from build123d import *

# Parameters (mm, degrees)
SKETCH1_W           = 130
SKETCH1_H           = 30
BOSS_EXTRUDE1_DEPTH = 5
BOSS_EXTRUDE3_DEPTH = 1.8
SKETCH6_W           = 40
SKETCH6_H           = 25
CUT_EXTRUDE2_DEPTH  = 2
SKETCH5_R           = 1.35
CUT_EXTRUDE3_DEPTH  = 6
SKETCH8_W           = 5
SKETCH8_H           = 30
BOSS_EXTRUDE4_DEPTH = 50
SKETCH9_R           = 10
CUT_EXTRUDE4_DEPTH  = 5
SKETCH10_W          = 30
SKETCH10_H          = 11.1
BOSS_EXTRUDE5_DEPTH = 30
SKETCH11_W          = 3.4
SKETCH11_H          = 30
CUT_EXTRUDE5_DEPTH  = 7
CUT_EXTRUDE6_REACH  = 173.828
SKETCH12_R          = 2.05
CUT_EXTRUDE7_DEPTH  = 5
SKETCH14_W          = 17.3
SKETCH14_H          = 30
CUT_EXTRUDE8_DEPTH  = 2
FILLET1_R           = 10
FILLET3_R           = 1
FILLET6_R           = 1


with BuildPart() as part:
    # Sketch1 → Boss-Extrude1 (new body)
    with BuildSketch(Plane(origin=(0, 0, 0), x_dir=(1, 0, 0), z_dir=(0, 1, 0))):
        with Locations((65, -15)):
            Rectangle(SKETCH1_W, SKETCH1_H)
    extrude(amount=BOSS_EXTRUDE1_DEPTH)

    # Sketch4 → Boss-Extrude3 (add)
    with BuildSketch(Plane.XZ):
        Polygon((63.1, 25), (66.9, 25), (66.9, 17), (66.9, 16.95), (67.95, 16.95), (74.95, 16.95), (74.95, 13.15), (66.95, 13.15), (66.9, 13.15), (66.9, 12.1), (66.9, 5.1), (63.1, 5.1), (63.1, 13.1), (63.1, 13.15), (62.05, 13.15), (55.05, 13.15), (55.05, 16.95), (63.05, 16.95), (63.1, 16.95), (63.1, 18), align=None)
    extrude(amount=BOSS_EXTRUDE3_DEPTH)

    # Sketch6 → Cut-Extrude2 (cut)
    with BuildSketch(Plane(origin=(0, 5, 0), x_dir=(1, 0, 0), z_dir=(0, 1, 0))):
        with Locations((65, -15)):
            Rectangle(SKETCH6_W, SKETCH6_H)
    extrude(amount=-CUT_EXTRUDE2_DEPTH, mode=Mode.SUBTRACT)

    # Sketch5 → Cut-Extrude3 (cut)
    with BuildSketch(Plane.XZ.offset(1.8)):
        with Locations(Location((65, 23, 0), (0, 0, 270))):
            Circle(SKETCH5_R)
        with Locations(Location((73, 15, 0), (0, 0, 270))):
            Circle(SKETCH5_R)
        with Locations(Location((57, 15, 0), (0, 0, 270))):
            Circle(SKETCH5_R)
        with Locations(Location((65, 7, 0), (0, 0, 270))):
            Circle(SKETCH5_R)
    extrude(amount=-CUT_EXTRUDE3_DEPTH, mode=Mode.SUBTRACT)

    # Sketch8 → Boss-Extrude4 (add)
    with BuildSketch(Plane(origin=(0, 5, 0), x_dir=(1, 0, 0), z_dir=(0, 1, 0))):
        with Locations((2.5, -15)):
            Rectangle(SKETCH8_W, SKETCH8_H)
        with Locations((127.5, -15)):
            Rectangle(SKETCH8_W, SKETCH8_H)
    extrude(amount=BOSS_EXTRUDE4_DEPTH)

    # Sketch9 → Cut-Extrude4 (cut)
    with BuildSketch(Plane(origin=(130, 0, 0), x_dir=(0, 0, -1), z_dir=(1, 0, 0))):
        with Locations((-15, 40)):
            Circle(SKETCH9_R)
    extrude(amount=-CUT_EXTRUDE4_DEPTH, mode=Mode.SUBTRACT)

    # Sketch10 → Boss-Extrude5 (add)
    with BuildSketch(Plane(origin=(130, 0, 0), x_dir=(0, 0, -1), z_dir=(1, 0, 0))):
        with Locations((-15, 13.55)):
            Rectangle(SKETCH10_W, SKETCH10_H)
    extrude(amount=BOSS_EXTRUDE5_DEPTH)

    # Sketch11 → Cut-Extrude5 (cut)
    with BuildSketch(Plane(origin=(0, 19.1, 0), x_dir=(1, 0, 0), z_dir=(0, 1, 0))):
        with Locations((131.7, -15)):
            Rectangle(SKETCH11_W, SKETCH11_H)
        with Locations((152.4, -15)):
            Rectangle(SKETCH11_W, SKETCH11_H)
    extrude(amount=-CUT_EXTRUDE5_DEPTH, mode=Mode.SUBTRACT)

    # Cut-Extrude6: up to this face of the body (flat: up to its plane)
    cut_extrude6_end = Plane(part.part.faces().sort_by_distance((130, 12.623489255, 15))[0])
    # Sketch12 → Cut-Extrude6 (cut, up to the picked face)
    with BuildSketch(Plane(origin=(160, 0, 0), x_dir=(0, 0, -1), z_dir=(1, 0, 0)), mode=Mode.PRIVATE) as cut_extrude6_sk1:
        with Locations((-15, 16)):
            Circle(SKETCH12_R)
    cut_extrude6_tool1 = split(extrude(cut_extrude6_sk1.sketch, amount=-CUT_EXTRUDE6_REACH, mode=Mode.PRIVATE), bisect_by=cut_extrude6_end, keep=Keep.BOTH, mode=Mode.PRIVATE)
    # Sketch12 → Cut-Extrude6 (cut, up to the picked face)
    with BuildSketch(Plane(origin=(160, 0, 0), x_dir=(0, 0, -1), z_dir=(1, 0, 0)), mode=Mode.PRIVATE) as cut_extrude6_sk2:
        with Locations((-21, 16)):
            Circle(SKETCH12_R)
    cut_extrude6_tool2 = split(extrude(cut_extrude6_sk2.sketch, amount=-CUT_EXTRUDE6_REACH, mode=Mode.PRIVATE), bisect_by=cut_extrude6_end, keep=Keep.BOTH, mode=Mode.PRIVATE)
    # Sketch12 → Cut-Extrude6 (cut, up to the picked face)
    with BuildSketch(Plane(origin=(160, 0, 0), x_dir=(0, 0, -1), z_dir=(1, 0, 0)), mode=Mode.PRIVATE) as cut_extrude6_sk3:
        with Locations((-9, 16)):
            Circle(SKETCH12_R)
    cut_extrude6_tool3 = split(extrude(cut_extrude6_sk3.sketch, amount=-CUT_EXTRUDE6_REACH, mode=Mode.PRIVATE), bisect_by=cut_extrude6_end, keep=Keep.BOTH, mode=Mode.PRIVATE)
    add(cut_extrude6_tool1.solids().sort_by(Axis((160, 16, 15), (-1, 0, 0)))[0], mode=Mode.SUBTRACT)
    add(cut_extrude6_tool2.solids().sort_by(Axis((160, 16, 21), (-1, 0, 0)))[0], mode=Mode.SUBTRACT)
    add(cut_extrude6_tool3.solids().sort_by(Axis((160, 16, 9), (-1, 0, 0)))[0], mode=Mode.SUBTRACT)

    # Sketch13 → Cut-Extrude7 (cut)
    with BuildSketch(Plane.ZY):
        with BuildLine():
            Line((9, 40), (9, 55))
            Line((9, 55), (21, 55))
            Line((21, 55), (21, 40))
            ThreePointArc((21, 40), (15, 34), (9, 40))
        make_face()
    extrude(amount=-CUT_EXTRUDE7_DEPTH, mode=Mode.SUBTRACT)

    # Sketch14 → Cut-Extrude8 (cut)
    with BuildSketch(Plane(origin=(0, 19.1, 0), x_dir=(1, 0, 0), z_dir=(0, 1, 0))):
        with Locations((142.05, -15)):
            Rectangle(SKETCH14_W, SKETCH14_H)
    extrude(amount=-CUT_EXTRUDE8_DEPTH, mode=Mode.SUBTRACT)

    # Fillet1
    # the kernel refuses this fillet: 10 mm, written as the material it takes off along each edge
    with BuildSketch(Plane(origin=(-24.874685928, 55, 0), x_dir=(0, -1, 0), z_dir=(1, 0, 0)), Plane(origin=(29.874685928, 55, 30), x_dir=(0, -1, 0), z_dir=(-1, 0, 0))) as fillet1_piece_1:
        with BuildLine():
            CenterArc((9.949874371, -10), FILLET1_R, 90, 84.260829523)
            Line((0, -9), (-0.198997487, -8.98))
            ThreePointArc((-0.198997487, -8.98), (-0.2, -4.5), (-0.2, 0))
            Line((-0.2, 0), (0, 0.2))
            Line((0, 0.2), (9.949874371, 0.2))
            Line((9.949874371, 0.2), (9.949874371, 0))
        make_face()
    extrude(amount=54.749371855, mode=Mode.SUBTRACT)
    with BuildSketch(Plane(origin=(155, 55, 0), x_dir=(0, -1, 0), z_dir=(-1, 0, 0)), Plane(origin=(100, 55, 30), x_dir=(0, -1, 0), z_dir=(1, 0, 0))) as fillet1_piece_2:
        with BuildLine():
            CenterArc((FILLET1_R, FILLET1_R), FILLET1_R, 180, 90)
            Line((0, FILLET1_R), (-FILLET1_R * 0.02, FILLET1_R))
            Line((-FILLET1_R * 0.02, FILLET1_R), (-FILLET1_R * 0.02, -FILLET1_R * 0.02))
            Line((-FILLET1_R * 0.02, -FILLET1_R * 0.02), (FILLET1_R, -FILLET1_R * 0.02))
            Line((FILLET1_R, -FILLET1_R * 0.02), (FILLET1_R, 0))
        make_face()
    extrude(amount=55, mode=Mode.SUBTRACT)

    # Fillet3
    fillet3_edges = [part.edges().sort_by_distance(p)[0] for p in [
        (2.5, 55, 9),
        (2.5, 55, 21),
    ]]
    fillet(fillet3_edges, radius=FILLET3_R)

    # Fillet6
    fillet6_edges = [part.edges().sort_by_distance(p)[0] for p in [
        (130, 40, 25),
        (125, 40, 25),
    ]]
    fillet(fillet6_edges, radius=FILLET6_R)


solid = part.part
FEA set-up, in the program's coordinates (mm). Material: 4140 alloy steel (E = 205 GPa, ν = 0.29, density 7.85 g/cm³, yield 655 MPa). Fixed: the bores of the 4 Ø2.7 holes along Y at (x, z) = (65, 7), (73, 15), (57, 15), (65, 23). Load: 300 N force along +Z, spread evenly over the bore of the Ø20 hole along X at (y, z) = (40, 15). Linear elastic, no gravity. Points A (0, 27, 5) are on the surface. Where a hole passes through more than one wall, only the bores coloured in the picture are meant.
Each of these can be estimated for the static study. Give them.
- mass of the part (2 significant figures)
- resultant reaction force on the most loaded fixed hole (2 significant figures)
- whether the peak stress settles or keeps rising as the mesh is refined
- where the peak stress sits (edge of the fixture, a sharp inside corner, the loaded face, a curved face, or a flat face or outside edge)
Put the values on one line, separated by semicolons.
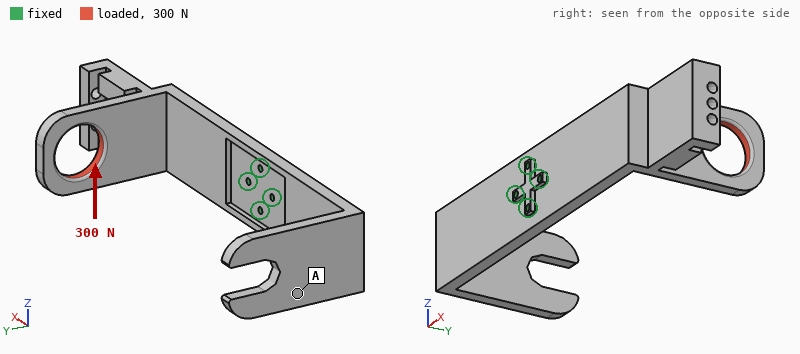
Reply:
280 g; 800 N; keeps rising; edge of the fixture
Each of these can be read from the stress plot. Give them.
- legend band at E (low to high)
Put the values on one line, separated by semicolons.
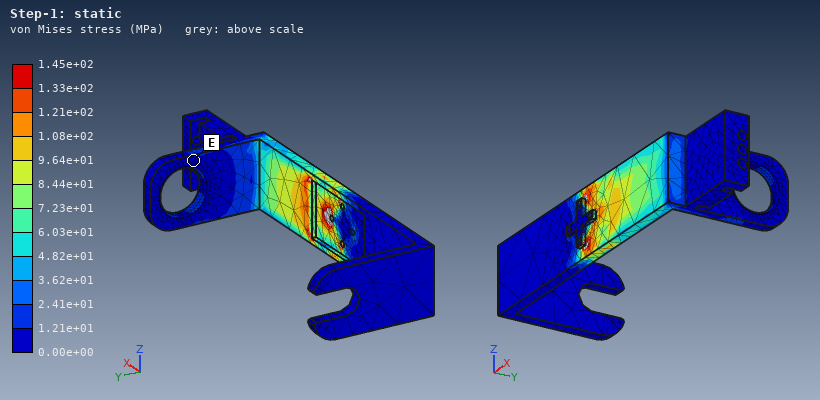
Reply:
0.00e+00 to 1.21e+01 MPa
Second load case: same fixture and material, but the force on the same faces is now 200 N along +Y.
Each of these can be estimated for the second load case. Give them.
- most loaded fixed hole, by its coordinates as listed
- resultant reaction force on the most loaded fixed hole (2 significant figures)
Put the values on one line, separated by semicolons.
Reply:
(73, 15); 900 N
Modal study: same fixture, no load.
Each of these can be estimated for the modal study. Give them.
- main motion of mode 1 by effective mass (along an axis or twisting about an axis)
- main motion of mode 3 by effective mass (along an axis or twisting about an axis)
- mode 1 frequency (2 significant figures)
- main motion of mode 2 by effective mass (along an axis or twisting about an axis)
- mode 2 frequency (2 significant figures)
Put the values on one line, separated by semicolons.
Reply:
along Y; along Z; 260 Hz; along Y; 390 Hz
